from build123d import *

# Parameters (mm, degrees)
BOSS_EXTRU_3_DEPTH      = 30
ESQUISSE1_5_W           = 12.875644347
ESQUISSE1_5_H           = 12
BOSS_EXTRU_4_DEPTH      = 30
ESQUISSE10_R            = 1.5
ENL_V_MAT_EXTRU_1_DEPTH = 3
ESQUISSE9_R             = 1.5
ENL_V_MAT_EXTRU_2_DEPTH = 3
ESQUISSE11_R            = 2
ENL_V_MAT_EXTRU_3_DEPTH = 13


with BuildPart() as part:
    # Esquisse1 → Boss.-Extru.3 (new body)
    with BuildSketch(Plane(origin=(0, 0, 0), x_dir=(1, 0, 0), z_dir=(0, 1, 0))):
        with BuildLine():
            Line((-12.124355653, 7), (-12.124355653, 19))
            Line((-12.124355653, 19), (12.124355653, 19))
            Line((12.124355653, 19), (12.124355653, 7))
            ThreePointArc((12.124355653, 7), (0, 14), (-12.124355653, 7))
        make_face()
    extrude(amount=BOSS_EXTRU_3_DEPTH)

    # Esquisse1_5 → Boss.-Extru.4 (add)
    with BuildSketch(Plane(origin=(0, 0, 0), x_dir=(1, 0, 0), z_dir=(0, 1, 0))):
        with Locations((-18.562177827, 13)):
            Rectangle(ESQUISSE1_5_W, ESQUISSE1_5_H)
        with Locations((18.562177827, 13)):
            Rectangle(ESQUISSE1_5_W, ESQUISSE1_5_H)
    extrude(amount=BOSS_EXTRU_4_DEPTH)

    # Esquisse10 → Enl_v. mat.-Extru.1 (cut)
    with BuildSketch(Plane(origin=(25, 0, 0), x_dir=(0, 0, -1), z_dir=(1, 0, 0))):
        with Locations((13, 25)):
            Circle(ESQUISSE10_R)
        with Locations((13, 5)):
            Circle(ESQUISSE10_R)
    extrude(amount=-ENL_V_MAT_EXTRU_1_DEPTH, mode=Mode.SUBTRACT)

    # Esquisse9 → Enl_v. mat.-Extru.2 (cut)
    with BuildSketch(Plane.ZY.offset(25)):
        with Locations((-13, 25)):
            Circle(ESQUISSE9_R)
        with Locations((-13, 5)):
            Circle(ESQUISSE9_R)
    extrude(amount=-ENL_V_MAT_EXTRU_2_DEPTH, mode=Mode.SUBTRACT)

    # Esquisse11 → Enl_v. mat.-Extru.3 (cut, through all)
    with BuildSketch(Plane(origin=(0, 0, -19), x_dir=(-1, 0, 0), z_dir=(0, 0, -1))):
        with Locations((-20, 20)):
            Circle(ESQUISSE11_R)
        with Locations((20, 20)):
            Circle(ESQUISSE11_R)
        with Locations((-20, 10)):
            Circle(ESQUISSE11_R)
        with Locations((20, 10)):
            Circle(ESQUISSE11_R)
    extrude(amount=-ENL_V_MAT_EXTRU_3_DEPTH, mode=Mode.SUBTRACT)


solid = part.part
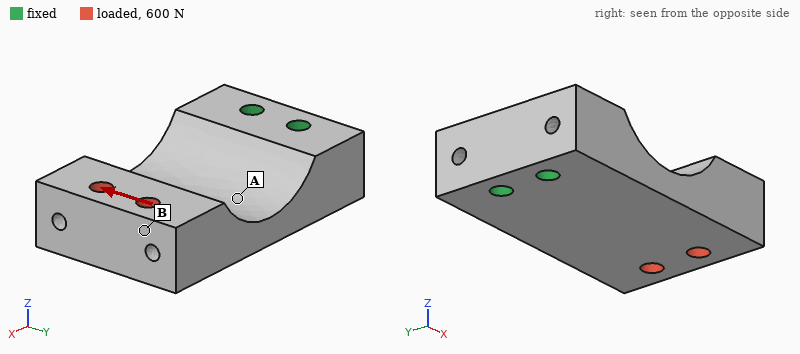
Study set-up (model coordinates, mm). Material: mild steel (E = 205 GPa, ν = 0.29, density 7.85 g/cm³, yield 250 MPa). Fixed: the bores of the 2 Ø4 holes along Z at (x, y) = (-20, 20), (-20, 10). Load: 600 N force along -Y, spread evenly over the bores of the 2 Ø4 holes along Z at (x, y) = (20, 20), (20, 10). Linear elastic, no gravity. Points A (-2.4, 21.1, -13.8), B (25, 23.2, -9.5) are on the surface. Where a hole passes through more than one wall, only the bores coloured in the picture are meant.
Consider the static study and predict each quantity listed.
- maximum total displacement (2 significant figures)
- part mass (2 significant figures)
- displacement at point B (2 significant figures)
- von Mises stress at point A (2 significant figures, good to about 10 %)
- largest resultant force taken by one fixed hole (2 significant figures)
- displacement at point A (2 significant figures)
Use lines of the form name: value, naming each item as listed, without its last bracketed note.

maximum total displacement: 12 µm
part mass: 110 g
displacement at point B: 11 µm
von Mises stress at point A: 20 MPa
largest resultant force taken by one fixed hole: 1.7 kN
displacement at point A: 2.9 µm
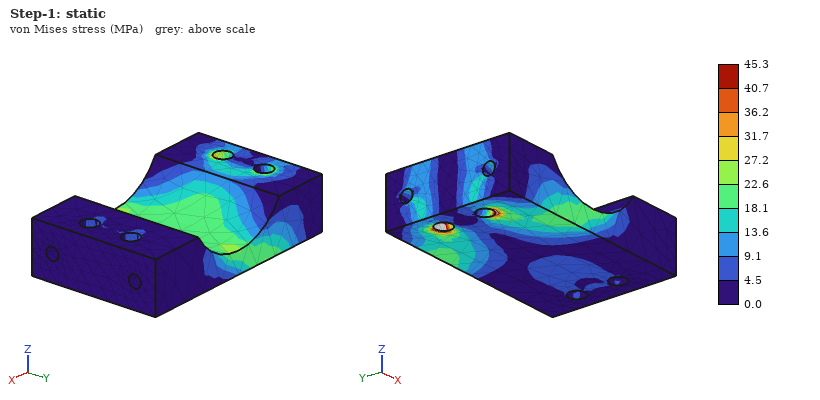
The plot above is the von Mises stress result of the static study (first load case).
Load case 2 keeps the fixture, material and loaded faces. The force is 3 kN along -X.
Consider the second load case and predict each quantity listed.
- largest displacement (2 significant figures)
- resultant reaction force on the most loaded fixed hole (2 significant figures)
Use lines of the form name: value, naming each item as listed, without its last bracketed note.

largest displacement: 53 µm
resultant reaction force on the most loaded fixed hole: 1.5 kN
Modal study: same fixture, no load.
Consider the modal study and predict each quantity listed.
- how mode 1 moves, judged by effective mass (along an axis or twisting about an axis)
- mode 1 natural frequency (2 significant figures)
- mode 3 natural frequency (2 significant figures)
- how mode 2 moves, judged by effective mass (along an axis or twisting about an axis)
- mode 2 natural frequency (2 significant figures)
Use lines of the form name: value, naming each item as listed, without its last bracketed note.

how mode 1 moves, judged by effective mass: along Z
mode 1 natural frequency: 2600 Hz
mode 3 natural frequency: 8400 Hz
how mode 2 moves, judged by effective mass: along Y
mode 2 natural frequency: 6100 Hz
